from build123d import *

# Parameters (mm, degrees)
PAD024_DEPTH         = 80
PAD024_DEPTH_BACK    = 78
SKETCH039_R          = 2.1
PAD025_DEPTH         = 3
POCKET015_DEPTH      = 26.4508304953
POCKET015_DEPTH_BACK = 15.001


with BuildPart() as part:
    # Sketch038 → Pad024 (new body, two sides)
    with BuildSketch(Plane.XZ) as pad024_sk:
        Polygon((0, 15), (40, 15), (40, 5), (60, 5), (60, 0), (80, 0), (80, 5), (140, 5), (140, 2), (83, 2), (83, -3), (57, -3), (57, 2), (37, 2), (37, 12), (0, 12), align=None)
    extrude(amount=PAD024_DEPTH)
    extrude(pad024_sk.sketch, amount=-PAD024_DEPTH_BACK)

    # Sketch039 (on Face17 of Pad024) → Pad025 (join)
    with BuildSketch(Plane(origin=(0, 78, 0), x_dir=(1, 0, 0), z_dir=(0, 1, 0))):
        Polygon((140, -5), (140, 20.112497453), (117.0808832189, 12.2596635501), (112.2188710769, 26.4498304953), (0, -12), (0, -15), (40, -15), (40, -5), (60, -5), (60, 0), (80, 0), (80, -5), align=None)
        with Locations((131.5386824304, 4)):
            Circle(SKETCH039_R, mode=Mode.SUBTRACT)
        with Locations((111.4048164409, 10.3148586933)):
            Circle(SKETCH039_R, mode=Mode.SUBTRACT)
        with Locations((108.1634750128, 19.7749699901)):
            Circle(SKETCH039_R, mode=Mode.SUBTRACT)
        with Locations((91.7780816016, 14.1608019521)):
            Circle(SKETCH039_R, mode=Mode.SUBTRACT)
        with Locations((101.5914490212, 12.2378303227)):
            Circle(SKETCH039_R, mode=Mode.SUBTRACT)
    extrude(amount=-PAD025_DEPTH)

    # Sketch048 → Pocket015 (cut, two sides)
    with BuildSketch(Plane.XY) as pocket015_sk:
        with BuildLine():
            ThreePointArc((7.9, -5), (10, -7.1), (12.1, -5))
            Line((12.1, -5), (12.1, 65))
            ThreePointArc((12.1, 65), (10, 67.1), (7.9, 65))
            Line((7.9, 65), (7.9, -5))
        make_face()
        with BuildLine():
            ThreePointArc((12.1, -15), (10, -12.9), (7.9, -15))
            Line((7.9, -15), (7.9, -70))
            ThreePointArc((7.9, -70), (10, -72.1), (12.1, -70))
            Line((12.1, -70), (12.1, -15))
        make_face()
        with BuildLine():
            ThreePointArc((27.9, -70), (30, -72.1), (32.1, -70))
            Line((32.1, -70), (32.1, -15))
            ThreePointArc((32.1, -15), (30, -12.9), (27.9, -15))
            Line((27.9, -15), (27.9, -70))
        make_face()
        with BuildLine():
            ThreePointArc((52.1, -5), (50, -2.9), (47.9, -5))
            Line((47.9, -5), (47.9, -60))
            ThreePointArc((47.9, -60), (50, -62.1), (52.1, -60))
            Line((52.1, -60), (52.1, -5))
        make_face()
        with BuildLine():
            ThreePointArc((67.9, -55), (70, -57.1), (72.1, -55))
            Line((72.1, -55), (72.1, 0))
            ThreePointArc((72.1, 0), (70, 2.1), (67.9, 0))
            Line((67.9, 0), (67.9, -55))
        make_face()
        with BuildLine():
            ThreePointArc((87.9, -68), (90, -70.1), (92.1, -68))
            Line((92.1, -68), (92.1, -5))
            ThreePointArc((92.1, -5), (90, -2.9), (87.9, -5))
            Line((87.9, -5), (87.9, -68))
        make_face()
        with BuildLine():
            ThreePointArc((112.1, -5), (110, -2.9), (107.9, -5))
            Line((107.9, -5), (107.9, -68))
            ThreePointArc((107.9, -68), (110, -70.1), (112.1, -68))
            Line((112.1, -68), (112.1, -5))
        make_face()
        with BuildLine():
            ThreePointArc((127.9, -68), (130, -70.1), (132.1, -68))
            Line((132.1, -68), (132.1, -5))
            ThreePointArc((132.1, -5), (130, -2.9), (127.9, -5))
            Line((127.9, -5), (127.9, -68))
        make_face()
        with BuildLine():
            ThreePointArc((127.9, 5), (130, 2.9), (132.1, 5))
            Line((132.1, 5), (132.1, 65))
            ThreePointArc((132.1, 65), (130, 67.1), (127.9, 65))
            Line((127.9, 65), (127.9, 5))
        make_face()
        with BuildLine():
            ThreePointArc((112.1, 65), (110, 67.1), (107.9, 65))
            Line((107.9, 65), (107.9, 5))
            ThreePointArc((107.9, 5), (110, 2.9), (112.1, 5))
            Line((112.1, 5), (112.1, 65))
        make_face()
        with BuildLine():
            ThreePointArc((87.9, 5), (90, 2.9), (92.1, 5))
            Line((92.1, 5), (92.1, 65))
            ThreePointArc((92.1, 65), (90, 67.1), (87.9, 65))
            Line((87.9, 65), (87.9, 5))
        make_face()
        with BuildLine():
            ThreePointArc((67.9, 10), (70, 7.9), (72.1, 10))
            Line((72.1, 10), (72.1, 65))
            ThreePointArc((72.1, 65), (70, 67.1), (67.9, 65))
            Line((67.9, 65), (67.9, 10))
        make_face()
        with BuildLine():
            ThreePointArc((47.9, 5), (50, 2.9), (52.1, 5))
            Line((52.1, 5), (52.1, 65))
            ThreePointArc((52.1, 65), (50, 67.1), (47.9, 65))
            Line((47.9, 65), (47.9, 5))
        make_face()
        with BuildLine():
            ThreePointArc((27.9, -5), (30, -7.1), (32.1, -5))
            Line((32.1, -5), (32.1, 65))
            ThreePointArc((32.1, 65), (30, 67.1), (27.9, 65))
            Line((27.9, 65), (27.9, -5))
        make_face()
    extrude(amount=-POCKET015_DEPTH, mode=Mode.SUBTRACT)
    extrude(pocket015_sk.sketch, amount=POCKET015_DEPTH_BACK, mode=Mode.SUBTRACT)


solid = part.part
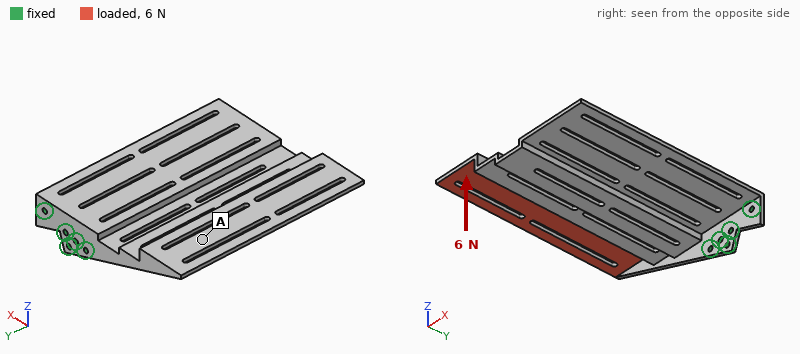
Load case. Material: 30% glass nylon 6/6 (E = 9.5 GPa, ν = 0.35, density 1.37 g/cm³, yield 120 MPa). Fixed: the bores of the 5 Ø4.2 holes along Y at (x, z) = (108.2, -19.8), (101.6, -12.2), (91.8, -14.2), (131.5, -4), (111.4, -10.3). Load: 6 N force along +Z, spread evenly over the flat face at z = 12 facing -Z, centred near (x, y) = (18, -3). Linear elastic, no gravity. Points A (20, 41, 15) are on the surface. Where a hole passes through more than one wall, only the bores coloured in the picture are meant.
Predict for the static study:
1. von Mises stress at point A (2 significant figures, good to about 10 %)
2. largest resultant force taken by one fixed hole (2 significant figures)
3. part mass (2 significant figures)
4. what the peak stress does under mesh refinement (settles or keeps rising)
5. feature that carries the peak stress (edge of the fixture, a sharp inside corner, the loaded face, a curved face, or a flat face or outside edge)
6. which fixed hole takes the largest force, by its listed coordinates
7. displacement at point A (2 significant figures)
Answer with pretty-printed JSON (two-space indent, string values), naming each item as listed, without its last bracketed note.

{
  "von Mises stress at point A": "1.2 MPa",
  "largest resultant force taken by one fixed hole": "26 N",
  "part mass": "96 g",
  "what the peak stress does under mesh refinement": "keeps rising",
  "feature that carries the peak stress": "edge of the fixture",
  "which fixed hole takes the largest force, by its listed coordinates": "(91.8, -14.2)",
  "displacement at point A": "0.66 mm"
}
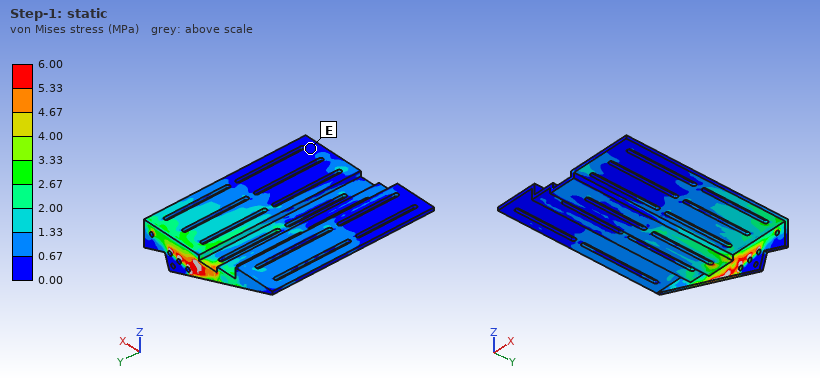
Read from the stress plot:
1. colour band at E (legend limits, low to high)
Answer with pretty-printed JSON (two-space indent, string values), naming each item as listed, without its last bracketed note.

{
  "colour band at E": "0.00 to 0.67 MPa"
}
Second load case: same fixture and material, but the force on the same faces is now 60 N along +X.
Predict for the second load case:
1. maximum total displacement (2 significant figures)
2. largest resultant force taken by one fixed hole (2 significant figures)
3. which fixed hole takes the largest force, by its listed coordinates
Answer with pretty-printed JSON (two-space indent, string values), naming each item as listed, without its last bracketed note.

{
  "maximum total displacement": "2.0 mm",
  "largest resultant force taken by one fixed hole": "140 N",
  "which fixed hole takes the largest force, by its listed coordinates": "(131.5, -4)"
}
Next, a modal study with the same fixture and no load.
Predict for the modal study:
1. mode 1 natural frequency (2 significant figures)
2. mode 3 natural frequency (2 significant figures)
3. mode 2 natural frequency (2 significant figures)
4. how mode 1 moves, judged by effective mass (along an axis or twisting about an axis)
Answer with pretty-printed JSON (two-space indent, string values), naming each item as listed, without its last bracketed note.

{
  "mode 1 natural frequency": "42 Hz",
  "mode 3 natural frequency": "170 Hz",
  "mode 2 natural frequency": "120 Hz",
  "how mode 1 moves, judged by effective mass": "along Z"
}
